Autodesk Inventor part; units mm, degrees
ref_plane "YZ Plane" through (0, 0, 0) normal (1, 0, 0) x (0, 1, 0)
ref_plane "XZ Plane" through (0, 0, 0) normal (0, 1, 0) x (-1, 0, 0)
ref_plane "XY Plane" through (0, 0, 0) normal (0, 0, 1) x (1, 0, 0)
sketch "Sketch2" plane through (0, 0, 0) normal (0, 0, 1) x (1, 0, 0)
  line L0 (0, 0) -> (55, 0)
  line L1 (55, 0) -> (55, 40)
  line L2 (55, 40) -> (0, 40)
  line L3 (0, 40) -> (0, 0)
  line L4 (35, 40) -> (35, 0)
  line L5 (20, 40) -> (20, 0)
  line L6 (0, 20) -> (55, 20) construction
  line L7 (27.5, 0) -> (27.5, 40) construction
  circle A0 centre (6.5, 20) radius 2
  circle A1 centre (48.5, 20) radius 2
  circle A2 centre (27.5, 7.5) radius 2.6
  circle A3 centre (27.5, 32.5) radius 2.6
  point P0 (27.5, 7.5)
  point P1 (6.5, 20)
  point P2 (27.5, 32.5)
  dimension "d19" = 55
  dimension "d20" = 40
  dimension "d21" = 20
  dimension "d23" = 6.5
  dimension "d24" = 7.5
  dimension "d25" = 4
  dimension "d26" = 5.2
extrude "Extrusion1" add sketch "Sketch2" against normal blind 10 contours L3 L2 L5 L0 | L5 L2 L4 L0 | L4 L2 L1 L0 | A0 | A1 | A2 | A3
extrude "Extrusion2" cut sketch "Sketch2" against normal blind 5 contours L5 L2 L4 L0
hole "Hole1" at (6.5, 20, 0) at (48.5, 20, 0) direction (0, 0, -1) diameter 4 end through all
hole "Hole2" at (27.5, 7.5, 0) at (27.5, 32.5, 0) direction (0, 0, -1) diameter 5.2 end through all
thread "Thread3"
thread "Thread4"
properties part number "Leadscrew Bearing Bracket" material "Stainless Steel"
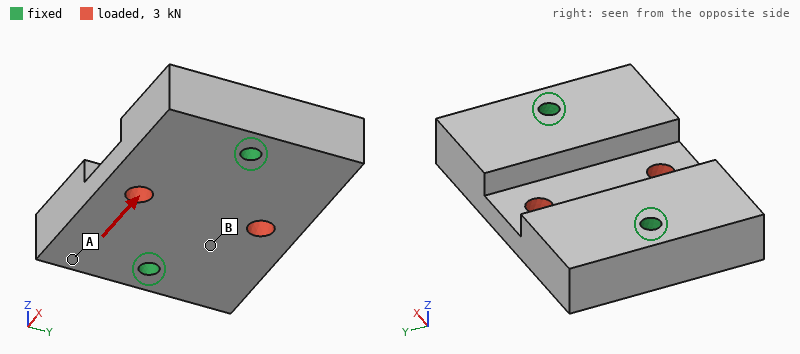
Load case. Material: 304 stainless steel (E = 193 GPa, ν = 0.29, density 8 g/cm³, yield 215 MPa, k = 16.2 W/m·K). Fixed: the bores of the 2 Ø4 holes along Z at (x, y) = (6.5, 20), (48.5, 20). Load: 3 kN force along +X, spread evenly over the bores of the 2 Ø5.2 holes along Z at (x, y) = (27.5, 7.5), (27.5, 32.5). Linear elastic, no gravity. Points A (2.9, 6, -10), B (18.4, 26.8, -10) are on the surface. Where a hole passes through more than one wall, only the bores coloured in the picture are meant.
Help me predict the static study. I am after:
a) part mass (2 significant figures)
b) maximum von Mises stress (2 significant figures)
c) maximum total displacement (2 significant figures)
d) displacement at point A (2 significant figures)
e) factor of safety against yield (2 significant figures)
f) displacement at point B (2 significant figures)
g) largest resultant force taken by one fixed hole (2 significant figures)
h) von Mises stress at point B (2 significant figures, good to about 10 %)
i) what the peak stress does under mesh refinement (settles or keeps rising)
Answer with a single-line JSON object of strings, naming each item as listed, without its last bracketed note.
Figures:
{"part mass": "150 g", "maximum von Mises stress": "34 MPa", "maximum total displacement": "1.8 µm", "displacement at point A": "0.93 µm", "factor of safety against yield": "6.4", "displacement at point B": "0.82 µm", "largest resultant force taken by one fixed hole": "1.5 kN", "von Mises stress at point B": "9.0 MPa", "what the peak stress does under mesh refinement": "settles"}
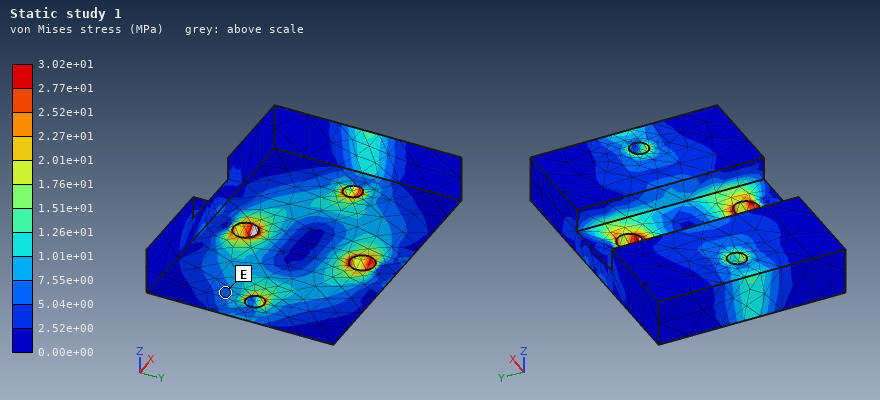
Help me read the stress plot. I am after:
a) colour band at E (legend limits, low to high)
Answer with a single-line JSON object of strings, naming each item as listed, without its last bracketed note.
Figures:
{"colour band at E": "5.04e+00 to 7.55e+00 MPa"}
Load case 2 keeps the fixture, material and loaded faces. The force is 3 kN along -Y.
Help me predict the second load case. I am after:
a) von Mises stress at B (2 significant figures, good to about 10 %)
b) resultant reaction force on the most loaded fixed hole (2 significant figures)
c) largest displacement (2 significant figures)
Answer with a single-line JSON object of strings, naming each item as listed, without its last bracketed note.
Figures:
{"von Mises stress at B": "18 MPa", "resultant reaction force on the most loaded fixed hole": "1.5 kN", "largest displacement": "4.6 µm"}
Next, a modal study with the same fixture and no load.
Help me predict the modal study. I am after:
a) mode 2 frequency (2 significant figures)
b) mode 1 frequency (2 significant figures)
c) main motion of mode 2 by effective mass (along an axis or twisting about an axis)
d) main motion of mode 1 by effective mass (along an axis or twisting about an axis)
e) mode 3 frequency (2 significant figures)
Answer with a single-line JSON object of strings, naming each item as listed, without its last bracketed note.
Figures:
{"mode 2 frequency": "14 kHz", "mode 1 frequency": "11 kHz", "main motion of mode 2 by effective mass": "along Z", "main motion of mode 1 by effective mass": "twisting about X", "mode 3 frequency": "16 kHz"}
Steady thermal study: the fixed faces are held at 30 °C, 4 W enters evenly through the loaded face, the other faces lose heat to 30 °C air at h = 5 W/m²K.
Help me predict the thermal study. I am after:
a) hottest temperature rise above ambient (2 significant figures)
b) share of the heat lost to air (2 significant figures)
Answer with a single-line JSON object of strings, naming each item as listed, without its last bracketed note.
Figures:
{"hottest temperature rise above ambient": "14 K", "share of the heat lost to air": "4.0 %"}
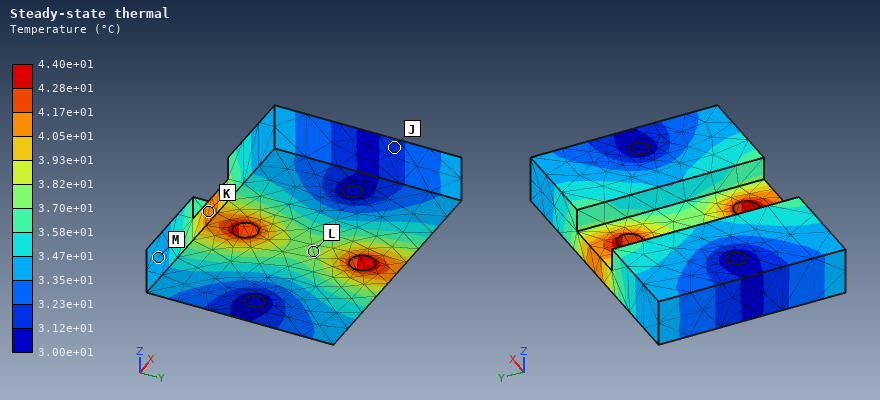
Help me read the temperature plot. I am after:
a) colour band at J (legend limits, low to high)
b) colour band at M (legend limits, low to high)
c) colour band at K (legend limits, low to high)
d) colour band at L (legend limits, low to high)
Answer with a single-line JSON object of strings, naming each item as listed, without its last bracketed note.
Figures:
{"colour band at J": "3.12e+01 to 3.23e+01 °C", "colour band at M": "3.35e+01 to 3.47e+01 °C", "colour band at K": "4.05e+01 to 4.17e+01 °C", "colour band at L": "3.70e+01 to 3.82e+01 °C"}
